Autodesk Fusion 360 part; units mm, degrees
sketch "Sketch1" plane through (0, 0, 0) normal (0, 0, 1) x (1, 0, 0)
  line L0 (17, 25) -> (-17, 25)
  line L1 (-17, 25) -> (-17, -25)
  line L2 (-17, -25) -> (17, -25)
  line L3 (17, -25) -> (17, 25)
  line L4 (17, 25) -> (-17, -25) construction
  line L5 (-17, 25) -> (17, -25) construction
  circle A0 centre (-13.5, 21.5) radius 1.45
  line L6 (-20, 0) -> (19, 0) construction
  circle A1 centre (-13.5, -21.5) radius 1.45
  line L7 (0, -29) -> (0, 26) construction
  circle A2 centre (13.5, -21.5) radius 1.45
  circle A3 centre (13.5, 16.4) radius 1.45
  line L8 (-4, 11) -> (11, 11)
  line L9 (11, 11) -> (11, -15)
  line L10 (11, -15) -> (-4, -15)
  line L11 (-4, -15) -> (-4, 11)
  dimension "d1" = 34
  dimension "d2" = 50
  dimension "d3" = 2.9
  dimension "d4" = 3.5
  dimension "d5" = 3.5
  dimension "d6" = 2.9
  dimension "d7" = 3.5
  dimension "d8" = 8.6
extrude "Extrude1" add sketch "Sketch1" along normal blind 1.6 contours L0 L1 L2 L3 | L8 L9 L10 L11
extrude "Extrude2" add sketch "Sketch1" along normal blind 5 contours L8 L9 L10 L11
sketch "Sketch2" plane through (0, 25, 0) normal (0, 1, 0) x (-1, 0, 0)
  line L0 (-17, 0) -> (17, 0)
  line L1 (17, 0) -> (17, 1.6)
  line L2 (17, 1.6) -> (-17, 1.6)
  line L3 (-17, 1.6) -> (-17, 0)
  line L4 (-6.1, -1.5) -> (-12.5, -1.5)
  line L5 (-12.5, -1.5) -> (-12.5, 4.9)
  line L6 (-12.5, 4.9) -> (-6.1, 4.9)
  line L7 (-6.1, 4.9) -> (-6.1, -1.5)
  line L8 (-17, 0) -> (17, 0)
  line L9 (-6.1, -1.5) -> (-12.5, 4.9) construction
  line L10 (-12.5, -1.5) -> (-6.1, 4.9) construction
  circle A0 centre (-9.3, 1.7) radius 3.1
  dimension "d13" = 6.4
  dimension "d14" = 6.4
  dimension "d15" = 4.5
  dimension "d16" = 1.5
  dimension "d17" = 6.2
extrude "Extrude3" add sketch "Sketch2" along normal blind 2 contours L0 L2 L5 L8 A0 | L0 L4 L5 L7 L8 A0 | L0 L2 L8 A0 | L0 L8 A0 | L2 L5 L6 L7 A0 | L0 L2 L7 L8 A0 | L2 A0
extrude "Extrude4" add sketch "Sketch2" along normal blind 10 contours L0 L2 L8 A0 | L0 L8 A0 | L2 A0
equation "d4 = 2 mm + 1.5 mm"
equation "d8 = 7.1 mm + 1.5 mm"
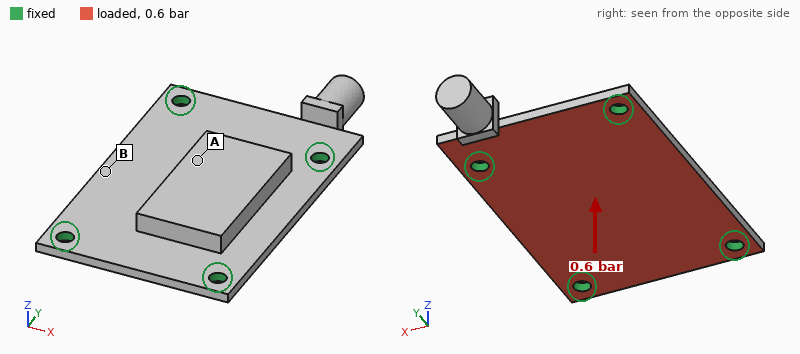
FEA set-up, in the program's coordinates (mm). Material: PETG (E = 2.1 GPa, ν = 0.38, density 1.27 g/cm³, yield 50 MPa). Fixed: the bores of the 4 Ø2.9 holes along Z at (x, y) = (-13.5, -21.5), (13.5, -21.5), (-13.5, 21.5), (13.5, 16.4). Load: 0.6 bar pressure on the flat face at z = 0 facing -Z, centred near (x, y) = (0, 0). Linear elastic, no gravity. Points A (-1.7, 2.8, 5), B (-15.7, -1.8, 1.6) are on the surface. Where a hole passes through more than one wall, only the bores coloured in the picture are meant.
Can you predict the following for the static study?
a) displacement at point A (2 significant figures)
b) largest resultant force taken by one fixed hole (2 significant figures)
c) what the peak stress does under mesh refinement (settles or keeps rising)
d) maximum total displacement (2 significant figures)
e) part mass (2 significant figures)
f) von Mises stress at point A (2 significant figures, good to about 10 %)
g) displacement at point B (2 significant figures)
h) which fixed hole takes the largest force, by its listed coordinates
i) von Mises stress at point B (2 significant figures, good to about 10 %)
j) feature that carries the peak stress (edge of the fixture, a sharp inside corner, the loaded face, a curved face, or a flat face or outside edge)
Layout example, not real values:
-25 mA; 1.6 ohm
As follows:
0.29 mm; 35 N; keeps rising; 0.53 mm; 5.5 g; 2.8 MPa; 0.50 mm; (13.5, 16.4); 6.9 MPa; edge of the fixture
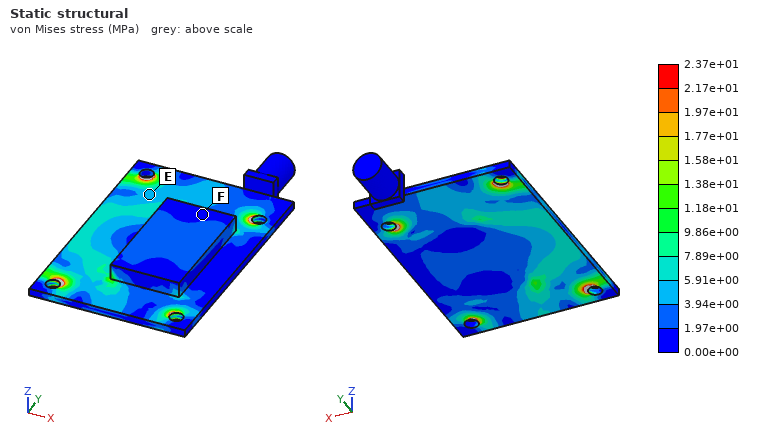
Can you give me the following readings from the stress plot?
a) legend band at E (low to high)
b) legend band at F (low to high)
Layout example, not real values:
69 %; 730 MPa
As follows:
3.94e+00 to 5.91e+00 MPa; 0.00e+00 to 1.97e+00 MPa
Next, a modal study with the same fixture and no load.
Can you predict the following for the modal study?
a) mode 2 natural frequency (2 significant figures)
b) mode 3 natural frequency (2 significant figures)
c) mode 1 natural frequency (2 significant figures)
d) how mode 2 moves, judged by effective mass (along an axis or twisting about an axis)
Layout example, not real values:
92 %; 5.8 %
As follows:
1300 Hz; 2300 Hz; 860 Hz; along Z
